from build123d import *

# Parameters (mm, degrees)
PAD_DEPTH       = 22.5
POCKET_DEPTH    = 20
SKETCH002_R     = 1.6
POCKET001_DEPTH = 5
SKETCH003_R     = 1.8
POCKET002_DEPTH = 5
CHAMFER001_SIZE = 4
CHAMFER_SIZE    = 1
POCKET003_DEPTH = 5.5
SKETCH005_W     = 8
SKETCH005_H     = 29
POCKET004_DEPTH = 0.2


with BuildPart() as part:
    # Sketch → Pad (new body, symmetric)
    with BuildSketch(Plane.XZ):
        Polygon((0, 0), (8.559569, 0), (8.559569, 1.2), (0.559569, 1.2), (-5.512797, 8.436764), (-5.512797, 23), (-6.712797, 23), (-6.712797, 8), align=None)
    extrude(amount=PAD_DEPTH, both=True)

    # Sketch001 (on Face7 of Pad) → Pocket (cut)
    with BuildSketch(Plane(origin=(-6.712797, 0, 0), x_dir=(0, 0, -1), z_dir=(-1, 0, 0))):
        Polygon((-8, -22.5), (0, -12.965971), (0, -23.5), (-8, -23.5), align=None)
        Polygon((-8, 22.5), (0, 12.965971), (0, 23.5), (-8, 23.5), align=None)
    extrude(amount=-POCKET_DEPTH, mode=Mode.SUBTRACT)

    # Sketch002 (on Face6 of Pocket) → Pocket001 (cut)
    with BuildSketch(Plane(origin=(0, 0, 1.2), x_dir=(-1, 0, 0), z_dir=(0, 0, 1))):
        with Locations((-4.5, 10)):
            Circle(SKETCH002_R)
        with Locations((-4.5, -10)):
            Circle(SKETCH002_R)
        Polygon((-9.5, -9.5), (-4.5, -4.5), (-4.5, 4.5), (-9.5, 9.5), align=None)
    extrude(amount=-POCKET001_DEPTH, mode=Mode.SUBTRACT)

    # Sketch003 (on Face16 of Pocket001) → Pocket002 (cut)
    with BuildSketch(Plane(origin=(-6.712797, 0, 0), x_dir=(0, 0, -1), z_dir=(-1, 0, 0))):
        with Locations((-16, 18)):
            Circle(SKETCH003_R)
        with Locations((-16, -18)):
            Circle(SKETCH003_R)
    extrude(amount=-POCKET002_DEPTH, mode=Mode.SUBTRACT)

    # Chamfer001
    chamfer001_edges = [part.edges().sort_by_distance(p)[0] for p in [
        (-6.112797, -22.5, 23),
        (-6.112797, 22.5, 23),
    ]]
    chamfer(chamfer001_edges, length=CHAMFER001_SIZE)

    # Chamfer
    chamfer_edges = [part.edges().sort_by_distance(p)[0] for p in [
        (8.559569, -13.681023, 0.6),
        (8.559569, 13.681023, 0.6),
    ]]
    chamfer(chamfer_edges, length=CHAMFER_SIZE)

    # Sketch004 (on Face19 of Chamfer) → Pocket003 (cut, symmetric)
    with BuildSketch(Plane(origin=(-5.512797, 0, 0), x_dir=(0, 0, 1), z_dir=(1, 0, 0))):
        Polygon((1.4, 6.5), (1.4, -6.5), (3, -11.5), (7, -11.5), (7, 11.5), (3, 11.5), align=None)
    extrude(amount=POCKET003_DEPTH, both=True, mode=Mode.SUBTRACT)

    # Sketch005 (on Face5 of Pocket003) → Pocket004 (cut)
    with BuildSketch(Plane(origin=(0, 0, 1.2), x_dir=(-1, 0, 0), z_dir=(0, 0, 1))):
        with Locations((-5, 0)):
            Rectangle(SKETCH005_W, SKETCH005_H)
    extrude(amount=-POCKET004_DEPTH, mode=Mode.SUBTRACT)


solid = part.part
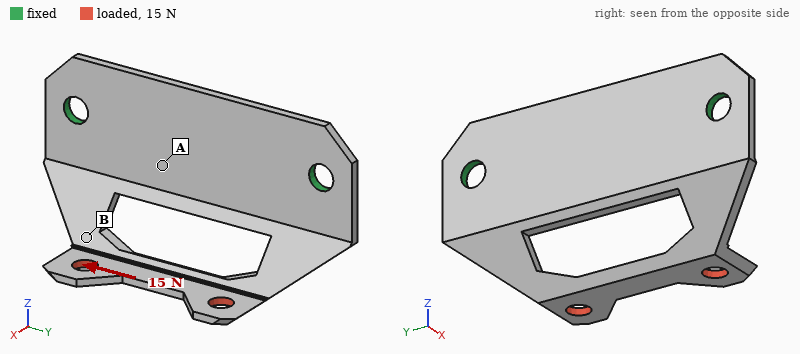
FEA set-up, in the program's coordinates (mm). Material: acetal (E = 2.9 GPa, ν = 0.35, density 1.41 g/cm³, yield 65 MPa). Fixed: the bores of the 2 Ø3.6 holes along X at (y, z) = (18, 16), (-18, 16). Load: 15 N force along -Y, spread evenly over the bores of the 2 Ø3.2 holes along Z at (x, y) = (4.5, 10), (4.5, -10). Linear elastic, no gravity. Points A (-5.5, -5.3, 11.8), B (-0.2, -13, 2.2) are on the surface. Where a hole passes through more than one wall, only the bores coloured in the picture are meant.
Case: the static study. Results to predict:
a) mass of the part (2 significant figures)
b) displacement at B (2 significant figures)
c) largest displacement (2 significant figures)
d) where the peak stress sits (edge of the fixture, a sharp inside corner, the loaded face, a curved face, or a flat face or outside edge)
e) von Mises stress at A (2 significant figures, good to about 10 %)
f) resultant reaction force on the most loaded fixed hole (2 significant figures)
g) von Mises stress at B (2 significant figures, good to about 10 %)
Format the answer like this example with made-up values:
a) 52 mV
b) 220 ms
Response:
a) 1.6 g
b) 0.29 mm
c) 0.54 mm
d) a flat face or outside edge
e) 2.0 MPa
f) 10 N
g) 6.3 MPa
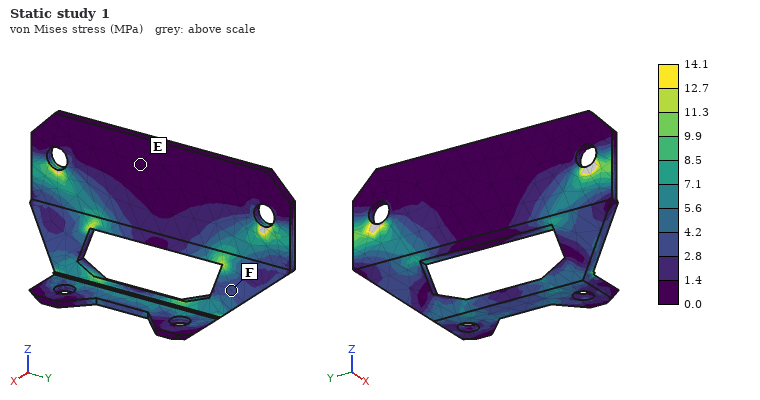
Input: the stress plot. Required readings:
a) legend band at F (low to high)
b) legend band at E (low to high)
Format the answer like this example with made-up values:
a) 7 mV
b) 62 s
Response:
a) 2.8 to 4.2 MPa
b) 0.0 to 1.4 MPa
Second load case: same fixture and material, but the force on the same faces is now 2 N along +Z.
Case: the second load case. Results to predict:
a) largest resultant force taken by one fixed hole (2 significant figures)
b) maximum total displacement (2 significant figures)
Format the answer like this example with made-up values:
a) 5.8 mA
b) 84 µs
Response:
a) 1.1 N
b) 0.62 mm
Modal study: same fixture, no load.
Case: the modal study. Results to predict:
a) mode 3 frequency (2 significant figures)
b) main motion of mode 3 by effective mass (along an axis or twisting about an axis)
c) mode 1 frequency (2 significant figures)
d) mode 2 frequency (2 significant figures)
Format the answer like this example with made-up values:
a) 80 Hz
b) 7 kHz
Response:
a) 1700 Hz
b) along X
c) 600 Hz
d) 1200 Hz
